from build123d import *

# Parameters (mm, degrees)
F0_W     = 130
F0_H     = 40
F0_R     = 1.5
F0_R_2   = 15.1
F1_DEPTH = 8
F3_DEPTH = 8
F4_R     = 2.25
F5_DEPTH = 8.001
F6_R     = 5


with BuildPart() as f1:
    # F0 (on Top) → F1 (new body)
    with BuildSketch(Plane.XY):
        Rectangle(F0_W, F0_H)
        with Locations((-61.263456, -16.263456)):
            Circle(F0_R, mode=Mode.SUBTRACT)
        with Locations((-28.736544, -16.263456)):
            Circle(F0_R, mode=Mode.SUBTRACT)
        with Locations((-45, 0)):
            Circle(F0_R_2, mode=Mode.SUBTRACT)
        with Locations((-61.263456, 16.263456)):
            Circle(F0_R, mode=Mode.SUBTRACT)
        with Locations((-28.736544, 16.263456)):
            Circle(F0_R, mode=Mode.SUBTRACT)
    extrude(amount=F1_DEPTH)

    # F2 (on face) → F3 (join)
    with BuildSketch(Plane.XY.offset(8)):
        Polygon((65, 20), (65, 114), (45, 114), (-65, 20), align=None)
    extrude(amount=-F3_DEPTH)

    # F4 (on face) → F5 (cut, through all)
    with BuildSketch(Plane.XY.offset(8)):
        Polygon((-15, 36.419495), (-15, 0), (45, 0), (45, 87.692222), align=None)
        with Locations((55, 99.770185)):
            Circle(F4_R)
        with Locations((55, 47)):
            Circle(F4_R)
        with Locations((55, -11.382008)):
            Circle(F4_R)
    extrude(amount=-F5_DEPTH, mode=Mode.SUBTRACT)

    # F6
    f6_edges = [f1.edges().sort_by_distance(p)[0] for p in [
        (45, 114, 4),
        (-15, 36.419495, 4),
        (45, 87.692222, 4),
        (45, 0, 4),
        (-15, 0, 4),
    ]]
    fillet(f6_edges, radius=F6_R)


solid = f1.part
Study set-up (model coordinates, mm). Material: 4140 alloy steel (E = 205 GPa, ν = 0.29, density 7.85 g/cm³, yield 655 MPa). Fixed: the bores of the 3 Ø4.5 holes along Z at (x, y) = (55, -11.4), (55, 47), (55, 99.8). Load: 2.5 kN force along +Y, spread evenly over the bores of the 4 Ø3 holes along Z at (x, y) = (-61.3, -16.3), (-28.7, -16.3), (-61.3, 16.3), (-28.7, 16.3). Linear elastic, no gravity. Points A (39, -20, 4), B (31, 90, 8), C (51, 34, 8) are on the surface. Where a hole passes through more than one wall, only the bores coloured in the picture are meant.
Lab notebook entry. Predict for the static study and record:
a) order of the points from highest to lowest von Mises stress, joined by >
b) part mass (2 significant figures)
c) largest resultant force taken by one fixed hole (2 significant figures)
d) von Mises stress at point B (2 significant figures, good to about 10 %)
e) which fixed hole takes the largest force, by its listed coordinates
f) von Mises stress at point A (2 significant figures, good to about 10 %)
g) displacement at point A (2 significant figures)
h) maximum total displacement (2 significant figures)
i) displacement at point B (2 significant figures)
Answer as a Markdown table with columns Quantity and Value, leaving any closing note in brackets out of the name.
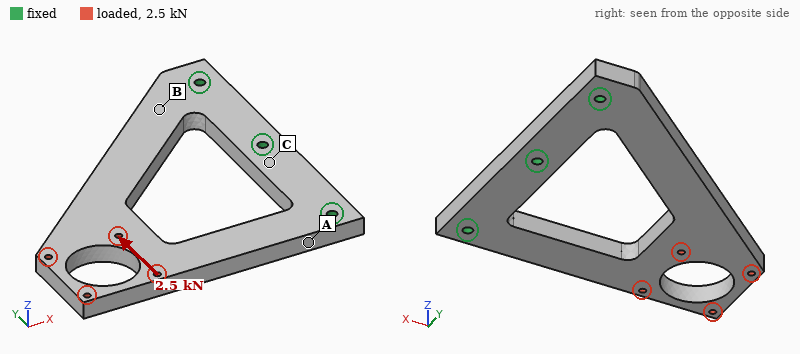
| Quantity | Value |
|---|---|
| order of the points from highest to lowest von Mises stress, joined by > | A > B > C |
| part mass | 490 g |
| largest resultant force taken by one fixed hole | 2.7 kN |
| von Mises stress at point B | 18 MPa |
| which fixed hole takes the largest force, by its listed coordinates | (55, 99.8) |
| von Mises stress at point A | 35 MPa |
| displacement at point A | 6.1 µm |
| maximum total displacement | 35 µm |
| displacement at point B | 7.2 µm |
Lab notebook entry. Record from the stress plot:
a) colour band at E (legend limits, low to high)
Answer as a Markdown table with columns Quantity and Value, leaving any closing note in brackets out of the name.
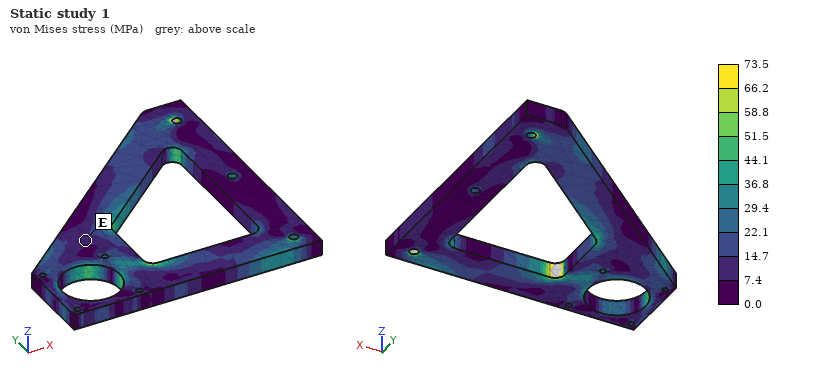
| Quantity | Value |
|---|---|
| colour band at E | 7.4 to 14.7 MPa |
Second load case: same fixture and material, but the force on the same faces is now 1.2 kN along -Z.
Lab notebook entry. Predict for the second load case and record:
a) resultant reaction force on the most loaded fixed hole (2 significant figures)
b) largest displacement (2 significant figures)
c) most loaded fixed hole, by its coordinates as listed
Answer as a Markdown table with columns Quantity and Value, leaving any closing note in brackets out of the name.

| Quantity | Value |
|---|---|
| resultant reaction force on the most loaded fixed hole | 1.1 kN |
| largest displacement | 1.7 mm |
| most loaded fixed hole, by its coordinates as listed | (55, -11.4) |
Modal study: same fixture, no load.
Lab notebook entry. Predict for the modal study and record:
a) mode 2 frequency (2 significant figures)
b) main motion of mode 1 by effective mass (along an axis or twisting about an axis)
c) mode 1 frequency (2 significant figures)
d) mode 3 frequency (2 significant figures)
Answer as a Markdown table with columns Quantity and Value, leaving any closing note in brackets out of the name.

| Quantity | Value |
|---|---|
| mode 2 frequency | 1600 Hz |
| main motion of mode 1 by effective mass | along Z |
| mode 1 frequency | 440 Hz |
| mode 3 frequency | 2500 Hz |
